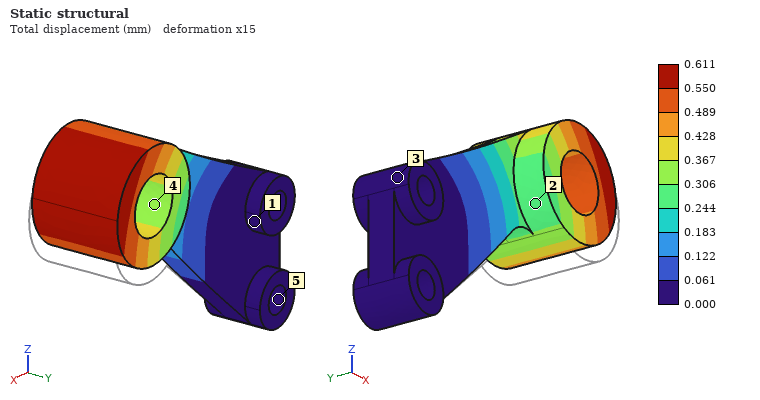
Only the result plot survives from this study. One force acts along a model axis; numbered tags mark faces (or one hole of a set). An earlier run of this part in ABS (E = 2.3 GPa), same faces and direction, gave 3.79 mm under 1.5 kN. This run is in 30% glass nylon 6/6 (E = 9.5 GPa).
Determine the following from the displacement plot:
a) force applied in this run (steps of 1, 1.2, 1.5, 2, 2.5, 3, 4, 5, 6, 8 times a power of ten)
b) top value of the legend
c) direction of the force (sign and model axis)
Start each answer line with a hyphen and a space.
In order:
- 1 kN
- 0.611 mm
- +Z
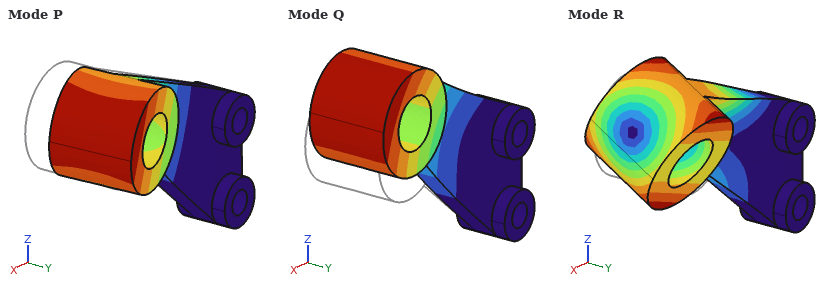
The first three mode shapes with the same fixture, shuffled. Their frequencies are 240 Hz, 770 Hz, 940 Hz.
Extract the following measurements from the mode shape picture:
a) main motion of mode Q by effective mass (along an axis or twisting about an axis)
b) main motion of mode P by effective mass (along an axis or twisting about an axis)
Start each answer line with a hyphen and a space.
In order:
- along Z
- along Y
